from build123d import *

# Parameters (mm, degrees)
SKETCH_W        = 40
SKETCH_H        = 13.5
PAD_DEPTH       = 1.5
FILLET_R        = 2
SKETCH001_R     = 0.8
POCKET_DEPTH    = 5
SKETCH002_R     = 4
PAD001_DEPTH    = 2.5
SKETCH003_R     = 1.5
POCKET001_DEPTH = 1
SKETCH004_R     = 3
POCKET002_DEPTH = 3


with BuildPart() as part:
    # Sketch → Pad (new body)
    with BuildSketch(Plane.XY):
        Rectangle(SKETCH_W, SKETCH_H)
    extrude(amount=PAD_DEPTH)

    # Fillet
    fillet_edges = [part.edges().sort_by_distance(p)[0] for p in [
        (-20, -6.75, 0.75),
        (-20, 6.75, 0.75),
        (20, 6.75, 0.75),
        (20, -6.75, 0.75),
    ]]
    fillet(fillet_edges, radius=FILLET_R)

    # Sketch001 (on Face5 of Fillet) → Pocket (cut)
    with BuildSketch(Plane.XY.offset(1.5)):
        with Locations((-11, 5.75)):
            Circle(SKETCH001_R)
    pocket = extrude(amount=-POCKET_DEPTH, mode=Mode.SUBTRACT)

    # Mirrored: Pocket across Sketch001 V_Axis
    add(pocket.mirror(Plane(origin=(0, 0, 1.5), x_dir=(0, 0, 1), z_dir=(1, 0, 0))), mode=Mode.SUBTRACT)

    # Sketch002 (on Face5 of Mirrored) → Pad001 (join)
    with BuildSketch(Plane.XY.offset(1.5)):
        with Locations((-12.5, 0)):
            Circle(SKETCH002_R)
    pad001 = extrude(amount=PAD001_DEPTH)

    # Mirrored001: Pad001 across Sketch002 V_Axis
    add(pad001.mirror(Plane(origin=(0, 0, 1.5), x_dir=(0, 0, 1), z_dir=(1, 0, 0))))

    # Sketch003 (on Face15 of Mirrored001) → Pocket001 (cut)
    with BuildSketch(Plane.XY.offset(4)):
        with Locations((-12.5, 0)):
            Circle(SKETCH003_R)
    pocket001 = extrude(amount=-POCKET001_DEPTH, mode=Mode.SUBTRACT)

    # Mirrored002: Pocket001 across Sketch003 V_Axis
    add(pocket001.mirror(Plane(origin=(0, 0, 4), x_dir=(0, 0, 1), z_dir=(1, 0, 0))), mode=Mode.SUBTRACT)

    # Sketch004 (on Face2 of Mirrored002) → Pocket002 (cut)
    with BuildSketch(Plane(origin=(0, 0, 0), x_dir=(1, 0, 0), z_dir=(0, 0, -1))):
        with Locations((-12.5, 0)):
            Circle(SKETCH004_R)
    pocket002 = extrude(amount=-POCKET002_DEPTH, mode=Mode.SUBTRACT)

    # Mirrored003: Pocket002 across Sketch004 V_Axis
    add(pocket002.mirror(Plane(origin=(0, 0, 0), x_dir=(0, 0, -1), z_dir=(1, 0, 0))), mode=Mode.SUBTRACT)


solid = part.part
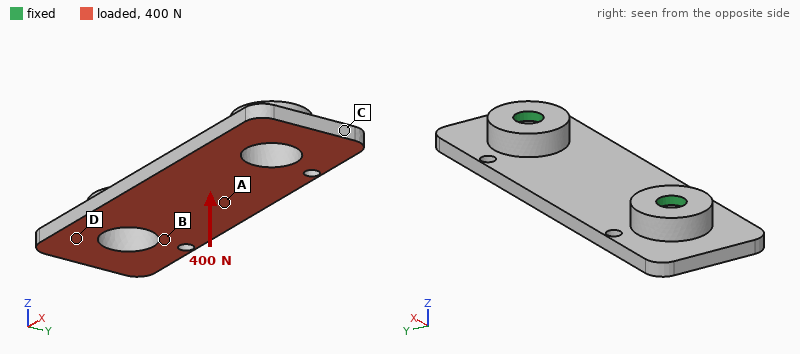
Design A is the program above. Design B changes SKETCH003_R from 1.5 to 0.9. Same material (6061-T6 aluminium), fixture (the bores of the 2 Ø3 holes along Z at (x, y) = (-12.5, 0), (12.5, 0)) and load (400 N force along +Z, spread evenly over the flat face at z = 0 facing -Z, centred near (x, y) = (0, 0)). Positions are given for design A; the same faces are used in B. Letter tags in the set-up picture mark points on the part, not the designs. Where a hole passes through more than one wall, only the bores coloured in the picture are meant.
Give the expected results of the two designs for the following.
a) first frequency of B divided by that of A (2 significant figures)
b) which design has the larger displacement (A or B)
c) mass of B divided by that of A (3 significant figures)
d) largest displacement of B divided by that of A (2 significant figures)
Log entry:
0.70
B
1.01
1.1
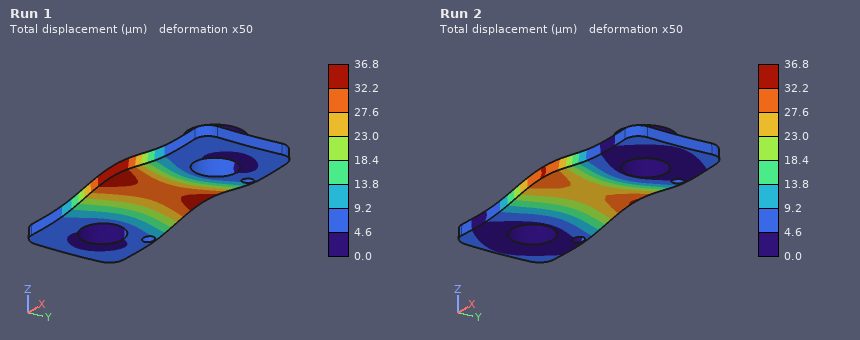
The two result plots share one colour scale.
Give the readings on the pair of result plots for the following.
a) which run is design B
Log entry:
Run 1
